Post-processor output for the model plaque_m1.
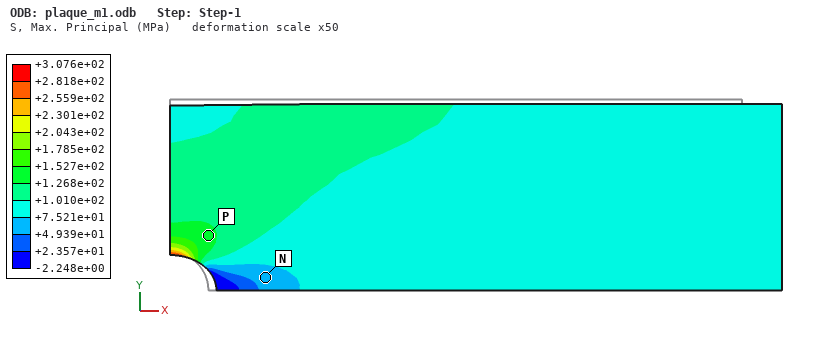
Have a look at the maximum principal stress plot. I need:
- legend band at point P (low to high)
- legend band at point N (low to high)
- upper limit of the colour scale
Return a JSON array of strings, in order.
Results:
["+1.268e+02 to +1.527e+02 MPa", "+4.939e+01 to +7.521e+01 MPa", "+3.076e+02 MPa"]
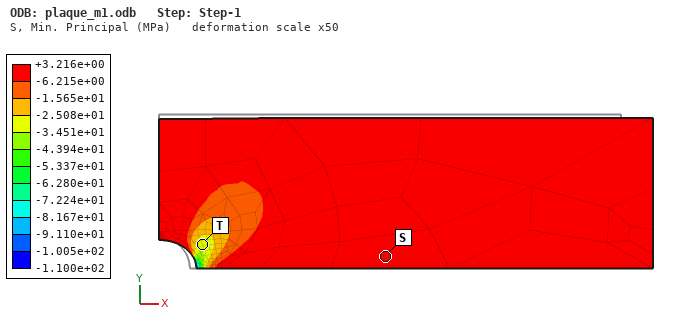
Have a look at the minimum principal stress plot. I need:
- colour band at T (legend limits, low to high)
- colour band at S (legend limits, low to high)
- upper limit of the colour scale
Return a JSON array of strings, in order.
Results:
["-3.451e+01 to -2.508e+01 MPa", "-6.215e+00 to +3.216e+00 MPa", "+3.216e+00 MPa"]
